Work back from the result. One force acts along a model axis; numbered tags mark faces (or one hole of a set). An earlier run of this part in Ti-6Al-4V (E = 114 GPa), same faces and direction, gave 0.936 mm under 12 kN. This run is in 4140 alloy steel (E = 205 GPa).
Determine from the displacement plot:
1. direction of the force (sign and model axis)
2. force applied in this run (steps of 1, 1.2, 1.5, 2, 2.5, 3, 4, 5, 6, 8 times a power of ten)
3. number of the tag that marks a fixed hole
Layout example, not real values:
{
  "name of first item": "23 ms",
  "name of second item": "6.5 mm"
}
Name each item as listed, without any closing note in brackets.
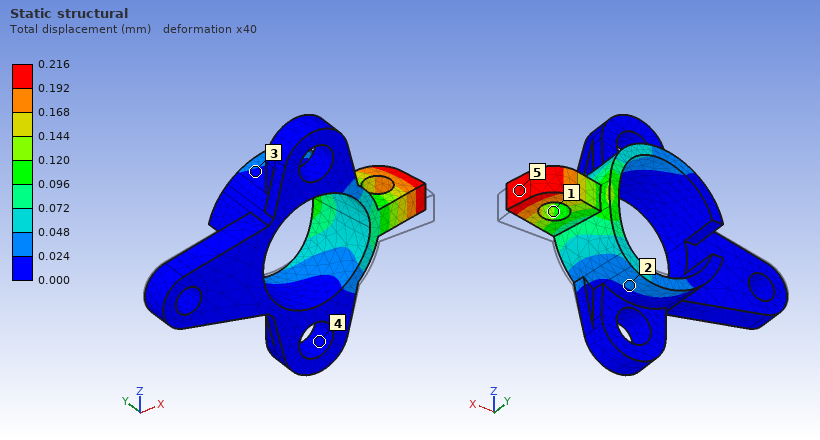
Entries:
{
  "direction of the force": "+Y",
  "force applied in this run": "5 kN",
  "number of the tag that marks a fixed hole": "4"
}
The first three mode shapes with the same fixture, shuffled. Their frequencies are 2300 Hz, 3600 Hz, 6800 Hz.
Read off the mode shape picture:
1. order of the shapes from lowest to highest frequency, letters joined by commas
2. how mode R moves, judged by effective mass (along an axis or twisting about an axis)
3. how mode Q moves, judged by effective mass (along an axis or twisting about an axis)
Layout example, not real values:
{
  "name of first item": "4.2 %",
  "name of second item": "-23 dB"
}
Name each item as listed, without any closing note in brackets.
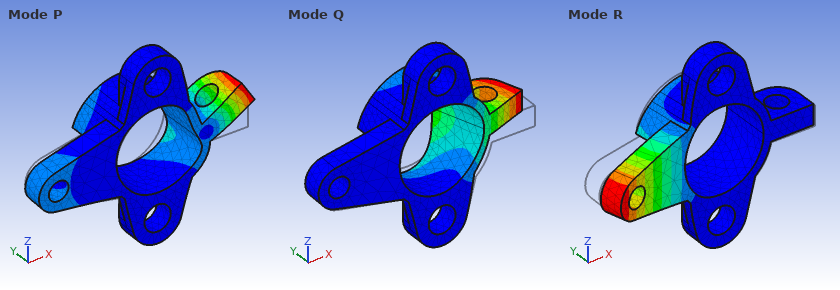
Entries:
{
  "order of the shapes from lowest to highest frequency, letters joined by commas": "R, Q, P",
  "how mode R moves, judged by effective mass": "along Y",
  "how mode Q moves, judged by effective mass": "along Y"
}
